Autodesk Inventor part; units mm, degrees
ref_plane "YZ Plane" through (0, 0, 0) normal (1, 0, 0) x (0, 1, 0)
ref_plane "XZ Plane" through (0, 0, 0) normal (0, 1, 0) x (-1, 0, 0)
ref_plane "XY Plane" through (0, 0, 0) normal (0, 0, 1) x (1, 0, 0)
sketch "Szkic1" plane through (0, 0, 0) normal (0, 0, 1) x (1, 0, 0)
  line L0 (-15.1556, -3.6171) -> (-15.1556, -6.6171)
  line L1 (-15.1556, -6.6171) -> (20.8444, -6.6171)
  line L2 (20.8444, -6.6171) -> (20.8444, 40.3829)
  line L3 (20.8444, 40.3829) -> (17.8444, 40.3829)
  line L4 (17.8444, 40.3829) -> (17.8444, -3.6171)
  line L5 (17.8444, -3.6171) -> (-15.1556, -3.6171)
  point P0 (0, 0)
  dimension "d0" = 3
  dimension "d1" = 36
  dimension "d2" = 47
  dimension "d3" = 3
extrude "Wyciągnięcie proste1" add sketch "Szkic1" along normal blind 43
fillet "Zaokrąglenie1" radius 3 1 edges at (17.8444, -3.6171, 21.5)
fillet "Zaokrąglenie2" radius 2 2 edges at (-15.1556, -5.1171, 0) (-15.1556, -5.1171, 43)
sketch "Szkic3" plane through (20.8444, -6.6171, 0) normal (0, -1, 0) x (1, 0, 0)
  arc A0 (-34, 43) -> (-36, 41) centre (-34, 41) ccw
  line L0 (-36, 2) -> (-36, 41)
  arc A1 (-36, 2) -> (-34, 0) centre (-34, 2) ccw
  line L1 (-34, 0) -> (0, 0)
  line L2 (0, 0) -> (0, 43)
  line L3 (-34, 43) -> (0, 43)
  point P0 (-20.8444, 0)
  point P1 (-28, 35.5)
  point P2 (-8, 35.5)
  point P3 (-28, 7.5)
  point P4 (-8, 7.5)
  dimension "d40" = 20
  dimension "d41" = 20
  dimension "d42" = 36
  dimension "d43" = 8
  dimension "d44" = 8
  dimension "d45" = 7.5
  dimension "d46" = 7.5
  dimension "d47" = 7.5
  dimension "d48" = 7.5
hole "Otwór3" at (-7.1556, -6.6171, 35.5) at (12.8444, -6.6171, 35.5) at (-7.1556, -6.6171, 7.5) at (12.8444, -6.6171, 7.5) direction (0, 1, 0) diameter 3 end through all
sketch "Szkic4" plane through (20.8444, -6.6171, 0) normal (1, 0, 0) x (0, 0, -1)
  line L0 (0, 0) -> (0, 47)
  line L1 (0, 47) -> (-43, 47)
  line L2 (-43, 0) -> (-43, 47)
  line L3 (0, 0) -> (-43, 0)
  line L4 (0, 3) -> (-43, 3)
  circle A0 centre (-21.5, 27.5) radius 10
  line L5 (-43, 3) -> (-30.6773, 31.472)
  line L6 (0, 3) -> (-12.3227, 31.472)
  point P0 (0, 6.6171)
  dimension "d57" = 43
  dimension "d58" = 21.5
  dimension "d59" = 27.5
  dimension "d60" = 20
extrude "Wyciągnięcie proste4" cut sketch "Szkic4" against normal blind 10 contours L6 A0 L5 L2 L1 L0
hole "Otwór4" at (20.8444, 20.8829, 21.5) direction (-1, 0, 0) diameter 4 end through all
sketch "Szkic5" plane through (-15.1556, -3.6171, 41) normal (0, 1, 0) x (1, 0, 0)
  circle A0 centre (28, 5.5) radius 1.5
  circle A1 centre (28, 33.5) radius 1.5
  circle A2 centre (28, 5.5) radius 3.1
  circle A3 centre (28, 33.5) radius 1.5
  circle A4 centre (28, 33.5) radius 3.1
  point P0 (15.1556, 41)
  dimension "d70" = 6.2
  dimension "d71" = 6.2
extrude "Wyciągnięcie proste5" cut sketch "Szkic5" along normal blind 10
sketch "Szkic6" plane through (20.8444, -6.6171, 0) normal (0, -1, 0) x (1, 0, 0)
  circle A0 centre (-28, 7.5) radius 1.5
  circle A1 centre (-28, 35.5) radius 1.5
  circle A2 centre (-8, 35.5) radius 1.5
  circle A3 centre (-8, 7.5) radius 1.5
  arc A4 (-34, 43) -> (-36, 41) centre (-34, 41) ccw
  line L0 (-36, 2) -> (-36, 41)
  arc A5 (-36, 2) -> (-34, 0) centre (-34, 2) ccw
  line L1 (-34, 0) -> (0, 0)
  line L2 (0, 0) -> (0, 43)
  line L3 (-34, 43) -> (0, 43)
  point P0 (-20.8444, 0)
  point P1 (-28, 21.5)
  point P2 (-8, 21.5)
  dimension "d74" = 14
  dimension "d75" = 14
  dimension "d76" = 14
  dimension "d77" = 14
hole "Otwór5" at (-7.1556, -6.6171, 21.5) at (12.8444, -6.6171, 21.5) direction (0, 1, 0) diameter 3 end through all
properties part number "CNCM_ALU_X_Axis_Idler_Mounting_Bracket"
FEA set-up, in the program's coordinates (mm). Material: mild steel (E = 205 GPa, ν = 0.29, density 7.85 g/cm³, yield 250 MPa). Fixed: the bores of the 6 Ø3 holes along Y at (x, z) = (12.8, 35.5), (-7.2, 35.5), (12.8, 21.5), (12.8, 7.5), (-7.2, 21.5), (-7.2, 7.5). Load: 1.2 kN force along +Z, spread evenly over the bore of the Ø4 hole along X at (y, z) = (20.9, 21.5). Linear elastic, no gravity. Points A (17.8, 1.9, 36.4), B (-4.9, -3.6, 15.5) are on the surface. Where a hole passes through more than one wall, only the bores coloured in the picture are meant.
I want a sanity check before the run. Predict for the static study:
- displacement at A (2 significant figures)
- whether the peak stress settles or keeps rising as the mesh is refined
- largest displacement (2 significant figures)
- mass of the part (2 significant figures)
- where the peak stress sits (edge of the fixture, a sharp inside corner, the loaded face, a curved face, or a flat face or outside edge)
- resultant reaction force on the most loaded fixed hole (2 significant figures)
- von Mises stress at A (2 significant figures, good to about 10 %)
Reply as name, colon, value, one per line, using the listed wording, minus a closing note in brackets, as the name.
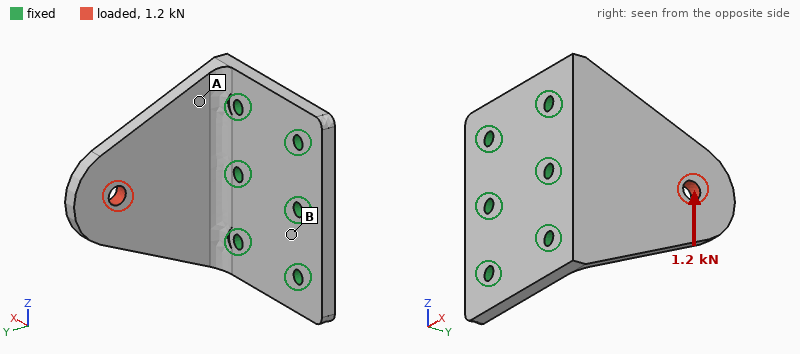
displacement at A: 15 µm
whether the peak stress settles or keeps rising as the mesh is refined: keeps rising
largest displacement: 34 µm
mass of the part: 58 g
where the peak stress sits: edge of the fixture
resultant reaction force on the most loaded fixed hole: 1.2 kN
von Mises stress at A: 72 MPa
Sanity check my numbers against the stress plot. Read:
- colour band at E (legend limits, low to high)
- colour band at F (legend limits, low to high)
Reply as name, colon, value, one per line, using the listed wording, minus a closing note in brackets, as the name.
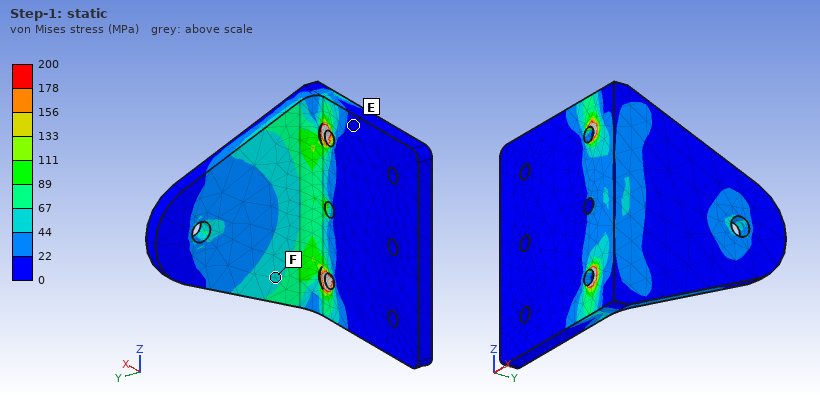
colour band at E: 0 to 22 MPa
colour band at F: 44 to 67 MPa
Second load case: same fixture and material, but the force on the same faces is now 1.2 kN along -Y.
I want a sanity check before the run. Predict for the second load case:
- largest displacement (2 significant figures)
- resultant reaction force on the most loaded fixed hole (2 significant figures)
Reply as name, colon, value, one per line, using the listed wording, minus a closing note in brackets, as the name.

largest displacement: 43 µm
resultant reaction force on the most loaded fixed hole: 440 N
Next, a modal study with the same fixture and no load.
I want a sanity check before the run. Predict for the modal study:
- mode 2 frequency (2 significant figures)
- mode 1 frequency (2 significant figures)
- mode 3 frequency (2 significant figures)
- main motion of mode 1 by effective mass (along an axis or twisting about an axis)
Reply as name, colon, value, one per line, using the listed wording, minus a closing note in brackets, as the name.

mode 2 frequency: 7800 Hz
mode 1 frequency: 2500 Hz
mode 3 frequency: 11 kHz
main motion of mode 1 by effective mass: along X
